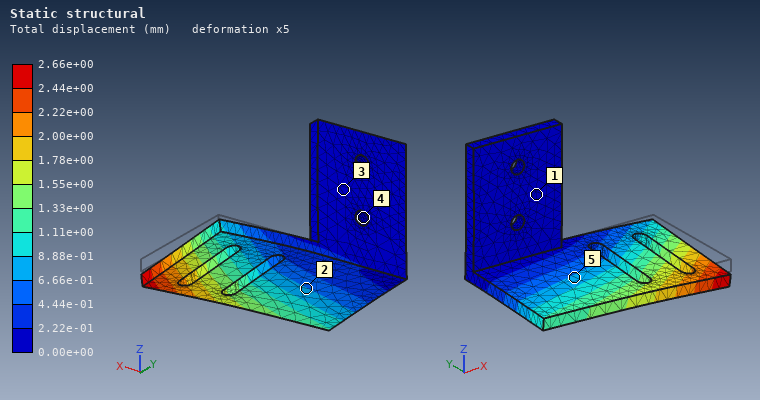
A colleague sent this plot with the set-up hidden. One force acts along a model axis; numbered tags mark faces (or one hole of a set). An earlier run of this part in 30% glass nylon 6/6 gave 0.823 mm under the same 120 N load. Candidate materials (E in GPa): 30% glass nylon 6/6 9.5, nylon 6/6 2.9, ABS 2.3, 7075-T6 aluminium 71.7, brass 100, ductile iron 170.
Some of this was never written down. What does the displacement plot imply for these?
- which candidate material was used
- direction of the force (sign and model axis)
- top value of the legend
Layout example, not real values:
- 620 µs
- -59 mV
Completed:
- nylon 6/6
- -Z
- 2.66e+00 mm
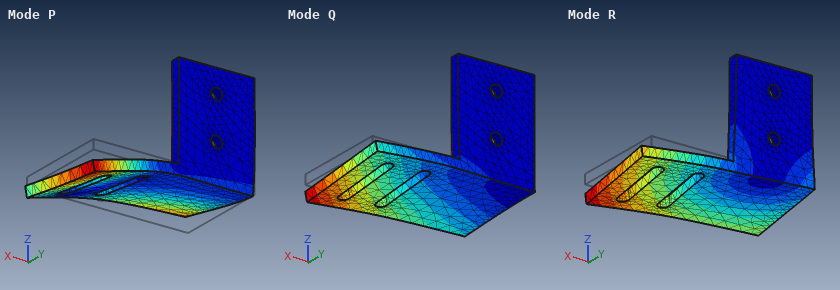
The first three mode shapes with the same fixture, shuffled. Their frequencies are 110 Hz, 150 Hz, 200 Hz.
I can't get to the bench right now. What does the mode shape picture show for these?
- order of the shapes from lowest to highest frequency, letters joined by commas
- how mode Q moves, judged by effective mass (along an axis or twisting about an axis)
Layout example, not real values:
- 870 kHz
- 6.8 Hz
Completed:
- Q, R, P
- along Z
